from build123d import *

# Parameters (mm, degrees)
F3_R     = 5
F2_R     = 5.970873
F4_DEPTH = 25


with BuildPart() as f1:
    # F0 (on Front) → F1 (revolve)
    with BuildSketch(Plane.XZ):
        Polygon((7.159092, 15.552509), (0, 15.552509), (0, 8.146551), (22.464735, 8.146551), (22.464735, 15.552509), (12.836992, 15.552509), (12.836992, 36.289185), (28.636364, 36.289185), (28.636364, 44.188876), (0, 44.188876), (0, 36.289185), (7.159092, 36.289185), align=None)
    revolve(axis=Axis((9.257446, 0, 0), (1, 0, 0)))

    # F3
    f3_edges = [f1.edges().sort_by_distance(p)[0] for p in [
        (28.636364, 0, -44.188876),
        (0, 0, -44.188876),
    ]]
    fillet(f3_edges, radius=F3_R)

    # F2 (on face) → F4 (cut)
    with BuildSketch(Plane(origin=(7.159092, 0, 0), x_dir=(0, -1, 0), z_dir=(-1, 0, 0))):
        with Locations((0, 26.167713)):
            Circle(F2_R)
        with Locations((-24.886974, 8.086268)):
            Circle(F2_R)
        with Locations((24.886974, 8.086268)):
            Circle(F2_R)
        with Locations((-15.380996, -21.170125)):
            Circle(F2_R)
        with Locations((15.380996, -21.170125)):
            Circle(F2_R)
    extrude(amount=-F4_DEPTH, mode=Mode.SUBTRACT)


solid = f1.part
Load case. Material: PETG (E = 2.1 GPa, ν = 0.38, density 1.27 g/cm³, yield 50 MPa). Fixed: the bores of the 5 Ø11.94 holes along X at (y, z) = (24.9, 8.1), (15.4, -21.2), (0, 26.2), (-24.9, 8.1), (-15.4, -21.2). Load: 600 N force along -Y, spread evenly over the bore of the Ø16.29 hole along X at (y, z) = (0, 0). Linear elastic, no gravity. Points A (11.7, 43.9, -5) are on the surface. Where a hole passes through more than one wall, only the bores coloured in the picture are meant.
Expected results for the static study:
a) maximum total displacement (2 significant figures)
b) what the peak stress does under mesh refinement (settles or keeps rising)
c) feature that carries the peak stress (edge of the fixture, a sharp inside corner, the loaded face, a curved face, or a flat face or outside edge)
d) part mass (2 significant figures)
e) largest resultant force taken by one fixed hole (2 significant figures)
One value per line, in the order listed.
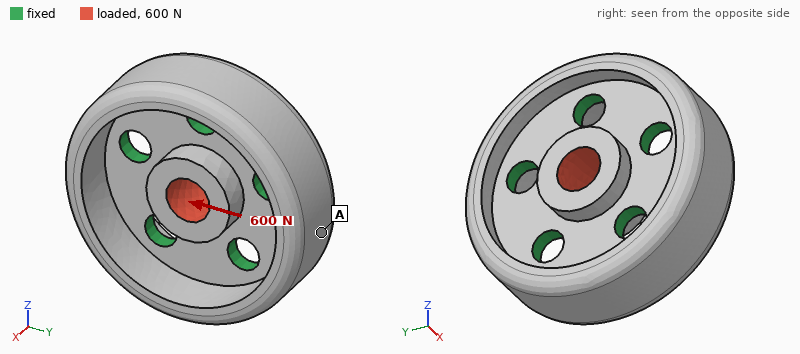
17 µm
keeps rising
edge of the fixture
100 g
170 N
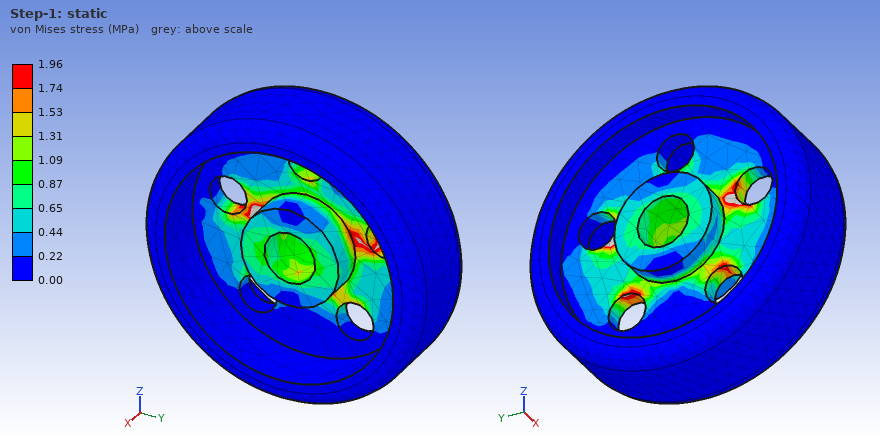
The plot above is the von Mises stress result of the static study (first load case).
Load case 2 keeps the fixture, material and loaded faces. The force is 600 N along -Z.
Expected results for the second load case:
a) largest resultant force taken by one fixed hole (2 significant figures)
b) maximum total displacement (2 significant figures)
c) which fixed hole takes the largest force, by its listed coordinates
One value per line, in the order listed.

180 N
17 µm
(0, 26.2)
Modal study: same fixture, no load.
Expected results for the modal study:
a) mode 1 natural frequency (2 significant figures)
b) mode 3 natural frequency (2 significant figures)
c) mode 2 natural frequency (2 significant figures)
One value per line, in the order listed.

2200 Hz
2600 Hz
2200 Hz
